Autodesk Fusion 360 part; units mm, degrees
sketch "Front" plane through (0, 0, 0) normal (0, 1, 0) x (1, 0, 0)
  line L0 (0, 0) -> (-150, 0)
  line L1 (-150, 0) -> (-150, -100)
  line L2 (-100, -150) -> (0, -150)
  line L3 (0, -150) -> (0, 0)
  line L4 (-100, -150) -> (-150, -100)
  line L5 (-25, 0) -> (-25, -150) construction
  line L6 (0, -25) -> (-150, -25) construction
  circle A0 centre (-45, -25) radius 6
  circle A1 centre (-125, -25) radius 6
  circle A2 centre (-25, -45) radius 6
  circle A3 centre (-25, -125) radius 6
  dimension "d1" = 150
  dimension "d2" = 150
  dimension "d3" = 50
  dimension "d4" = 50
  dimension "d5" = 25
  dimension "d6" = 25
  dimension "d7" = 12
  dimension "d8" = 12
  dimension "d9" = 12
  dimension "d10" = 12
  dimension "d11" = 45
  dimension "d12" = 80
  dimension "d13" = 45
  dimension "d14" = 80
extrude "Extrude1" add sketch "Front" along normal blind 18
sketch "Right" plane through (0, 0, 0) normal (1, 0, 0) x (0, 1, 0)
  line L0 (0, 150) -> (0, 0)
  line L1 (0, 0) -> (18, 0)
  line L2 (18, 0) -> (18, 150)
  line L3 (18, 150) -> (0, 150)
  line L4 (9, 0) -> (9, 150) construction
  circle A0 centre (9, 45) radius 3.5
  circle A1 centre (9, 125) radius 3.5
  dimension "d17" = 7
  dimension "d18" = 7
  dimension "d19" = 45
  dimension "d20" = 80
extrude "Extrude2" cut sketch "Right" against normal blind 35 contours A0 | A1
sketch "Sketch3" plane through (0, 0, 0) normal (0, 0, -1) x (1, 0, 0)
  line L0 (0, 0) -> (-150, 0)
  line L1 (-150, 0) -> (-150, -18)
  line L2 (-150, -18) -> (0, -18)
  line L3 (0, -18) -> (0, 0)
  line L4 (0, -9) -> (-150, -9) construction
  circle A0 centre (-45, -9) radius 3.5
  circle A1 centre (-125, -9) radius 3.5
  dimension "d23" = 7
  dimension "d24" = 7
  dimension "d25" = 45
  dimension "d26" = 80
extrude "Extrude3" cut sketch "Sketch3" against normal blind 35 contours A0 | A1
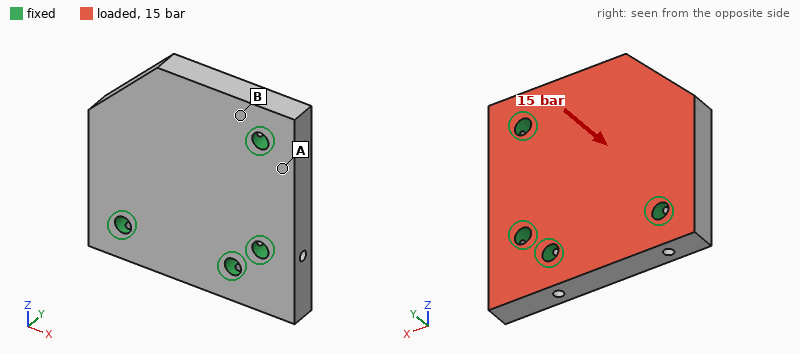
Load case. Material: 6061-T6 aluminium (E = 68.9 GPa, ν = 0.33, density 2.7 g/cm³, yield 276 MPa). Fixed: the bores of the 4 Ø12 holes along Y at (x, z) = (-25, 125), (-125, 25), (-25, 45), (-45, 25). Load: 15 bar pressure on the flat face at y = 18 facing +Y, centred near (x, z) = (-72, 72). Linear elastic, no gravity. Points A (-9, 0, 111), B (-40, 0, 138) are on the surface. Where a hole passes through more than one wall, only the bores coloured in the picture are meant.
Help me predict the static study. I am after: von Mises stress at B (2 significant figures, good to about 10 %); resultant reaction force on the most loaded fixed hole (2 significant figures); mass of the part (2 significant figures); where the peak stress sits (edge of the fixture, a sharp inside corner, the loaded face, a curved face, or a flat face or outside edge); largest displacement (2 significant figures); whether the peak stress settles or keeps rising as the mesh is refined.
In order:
46 MPa
11 kN
1.0 kg
edge of the fixture
0.24 mm
keeps rising
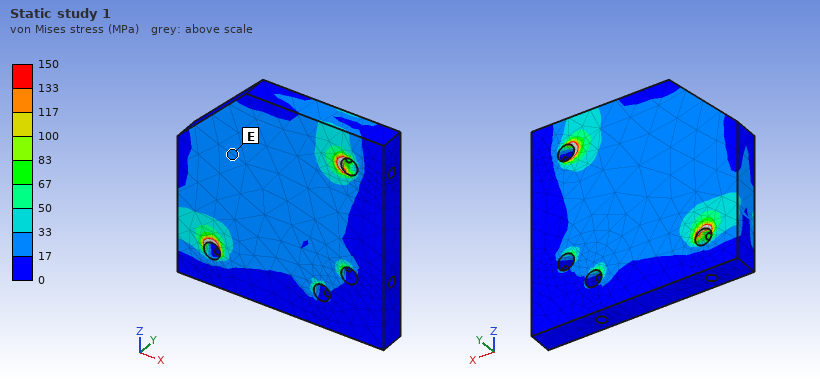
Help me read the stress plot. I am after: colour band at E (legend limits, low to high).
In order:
17 to 33 MPa
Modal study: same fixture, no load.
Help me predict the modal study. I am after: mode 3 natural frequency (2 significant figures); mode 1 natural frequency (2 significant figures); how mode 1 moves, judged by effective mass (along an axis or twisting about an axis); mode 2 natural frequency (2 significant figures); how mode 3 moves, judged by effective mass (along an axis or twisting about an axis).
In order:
7400 Hz
2400 Hz
along Y
5800 Hz
along Y
